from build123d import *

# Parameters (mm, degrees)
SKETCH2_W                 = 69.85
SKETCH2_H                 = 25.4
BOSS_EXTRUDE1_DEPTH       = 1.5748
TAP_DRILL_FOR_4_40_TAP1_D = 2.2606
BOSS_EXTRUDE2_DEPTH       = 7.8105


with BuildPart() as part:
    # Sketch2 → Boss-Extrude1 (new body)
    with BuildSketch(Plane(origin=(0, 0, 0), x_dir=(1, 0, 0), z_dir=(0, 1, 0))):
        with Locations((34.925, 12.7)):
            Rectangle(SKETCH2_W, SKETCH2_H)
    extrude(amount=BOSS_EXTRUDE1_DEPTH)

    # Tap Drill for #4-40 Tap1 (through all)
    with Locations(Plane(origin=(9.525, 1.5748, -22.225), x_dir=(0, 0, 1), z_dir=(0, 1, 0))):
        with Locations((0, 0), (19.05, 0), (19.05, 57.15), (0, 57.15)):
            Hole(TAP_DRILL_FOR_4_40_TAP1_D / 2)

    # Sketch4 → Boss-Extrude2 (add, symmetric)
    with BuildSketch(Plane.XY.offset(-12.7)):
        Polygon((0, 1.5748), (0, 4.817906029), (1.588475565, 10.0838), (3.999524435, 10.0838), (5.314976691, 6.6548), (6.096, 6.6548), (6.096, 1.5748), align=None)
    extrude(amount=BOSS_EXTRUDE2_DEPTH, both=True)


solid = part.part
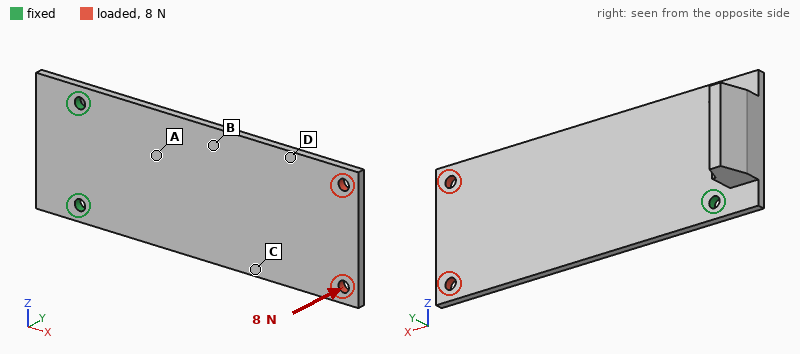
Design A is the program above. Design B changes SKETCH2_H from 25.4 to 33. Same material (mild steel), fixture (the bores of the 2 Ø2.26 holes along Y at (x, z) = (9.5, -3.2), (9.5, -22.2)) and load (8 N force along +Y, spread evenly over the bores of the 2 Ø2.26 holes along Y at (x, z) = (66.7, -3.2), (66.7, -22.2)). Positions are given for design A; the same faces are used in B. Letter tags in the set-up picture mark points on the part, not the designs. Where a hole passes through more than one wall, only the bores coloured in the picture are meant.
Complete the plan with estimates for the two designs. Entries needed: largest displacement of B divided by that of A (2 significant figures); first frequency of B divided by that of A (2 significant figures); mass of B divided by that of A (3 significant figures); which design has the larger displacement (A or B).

0.77
1.0
1.24
A
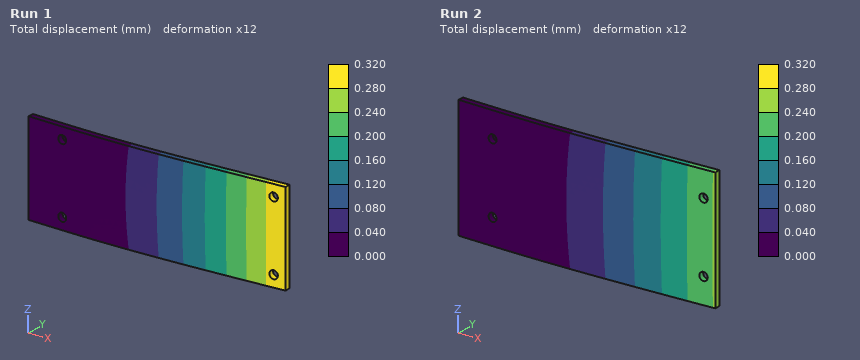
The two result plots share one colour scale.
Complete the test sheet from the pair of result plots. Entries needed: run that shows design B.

Run 2
